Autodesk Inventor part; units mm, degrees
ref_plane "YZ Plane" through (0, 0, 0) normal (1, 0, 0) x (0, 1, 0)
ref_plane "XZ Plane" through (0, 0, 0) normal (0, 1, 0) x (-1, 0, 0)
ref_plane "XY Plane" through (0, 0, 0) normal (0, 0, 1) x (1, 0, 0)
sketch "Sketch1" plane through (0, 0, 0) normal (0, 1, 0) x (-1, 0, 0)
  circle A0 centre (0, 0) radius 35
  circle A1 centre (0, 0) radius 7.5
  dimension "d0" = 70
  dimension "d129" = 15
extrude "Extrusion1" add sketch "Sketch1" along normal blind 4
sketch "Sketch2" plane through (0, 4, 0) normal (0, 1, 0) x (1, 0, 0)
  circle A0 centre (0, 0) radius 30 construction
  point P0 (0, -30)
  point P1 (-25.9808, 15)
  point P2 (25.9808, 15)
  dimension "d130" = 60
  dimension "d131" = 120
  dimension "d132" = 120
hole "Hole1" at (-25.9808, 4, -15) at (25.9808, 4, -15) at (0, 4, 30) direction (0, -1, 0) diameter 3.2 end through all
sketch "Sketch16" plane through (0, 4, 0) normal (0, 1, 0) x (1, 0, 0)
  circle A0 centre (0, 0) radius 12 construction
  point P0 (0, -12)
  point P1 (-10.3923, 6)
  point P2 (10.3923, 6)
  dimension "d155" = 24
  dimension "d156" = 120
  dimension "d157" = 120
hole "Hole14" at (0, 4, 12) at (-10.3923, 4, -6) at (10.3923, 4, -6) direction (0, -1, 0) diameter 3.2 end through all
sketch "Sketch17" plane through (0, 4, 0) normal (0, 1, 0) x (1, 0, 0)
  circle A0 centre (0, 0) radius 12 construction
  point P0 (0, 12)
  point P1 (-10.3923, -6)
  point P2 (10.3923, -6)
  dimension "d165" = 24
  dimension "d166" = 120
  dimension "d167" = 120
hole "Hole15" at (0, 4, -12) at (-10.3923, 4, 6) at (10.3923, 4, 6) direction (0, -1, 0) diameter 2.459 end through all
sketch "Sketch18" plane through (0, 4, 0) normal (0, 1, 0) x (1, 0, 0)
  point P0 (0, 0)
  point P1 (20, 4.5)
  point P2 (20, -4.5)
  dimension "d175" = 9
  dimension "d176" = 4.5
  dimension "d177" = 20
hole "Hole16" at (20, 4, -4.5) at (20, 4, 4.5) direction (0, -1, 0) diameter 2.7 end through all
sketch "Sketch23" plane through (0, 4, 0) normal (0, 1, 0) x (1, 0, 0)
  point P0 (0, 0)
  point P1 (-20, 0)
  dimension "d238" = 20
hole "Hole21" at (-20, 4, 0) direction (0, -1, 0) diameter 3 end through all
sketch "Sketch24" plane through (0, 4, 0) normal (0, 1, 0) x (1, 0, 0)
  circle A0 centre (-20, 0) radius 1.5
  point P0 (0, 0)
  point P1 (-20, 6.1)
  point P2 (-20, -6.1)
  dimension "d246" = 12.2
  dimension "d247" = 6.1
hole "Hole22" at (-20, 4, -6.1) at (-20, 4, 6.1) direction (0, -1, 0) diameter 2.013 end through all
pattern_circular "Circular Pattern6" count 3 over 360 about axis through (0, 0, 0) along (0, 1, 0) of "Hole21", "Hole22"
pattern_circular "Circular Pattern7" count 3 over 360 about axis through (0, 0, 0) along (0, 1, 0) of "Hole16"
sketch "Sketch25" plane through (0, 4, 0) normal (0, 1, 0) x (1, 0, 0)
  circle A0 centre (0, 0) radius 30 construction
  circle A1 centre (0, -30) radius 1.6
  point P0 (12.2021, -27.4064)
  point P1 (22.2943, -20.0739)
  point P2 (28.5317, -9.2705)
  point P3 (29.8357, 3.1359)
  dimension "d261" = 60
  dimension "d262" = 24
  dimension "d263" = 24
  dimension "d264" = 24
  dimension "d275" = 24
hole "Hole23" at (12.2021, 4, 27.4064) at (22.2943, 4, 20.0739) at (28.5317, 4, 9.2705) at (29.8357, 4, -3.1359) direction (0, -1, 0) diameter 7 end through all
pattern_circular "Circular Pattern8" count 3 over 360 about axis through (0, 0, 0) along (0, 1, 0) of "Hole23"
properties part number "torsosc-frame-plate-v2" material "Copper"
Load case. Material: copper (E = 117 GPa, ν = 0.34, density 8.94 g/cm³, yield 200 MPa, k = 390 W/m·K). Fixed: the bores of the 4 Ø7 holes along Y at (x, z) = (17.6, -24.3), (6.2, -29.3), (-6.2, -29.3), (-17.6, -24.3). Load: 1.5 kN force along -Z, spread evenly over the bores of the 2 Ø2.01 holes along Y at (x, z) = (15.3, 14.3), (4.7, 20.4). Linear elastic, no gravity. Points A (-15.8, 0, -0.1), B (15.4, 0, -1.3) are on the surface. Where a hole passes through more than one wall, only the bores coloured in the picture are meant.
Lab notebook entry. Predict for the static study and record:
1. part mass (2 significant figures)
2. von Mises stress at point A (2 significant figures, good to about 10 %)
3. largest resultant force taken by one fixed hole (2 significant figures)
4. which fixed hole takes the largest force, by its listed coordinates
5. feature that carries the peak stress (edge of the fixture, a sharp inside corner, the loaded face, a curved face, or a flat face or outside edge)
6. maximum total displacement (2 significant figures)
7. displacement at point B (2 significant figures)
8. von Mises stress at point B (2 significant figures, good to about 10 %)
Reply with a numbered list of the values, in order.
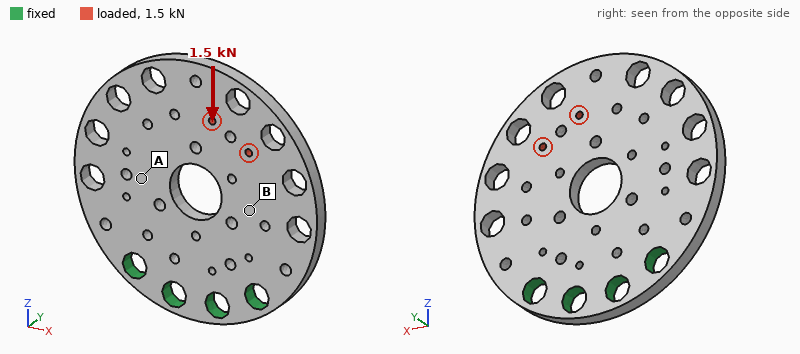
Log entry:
1. 110 g
2. 5.0 MPa
3. 950 N
4. (17.6, -24.3)
5. the loaded face
6. 7.0 µm
7. 3.7 µm
8. 19 MPa
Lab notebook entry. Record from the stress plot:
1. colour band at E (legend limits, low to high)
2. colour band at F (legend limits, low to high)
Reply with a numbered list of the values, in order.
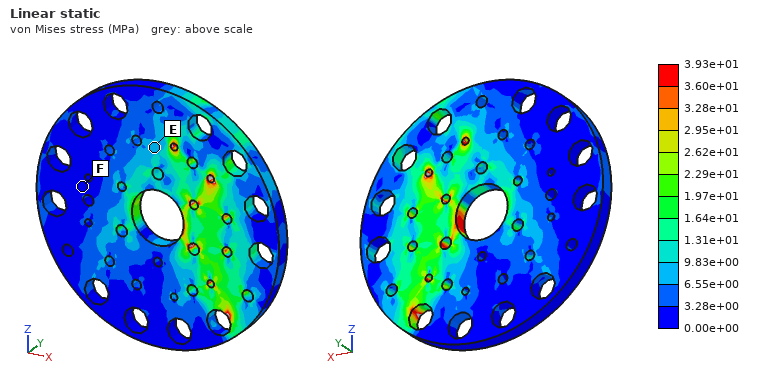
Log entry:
1. 6.55e+00 to 9.83e+00 MPa
2. 0.00e+00 to 3.28e+00 MPa
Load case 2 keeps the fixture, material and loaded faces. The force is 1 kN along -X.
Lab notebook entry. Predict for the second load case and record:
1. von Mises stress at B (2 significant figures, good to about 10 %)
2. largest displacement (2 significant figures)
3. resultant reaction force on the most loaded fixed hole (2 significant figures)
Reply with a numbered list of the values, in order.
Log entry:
1. 16 MPa
2. 16 µm
3. 1.0 kN
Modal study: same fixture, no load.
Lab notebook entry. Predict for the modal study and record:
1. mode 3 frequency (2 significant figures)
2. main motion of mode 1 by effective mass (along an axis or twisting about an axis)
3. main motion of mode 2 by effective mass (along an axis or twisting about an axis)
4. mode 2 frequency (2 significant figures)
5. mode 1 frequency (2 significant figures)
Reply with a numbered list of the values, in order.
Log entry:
1. 3800 Hz
2. along Y
3. twisting about Z
4. 1900 Hz
5. 810 Hz
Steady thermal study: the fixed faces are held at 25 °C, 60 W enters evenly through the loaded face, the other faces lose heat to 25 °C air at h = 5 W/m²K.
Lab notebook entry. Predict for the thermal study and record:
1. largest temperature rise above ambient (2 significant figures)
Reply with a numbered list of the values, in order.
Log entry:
1. 45 K
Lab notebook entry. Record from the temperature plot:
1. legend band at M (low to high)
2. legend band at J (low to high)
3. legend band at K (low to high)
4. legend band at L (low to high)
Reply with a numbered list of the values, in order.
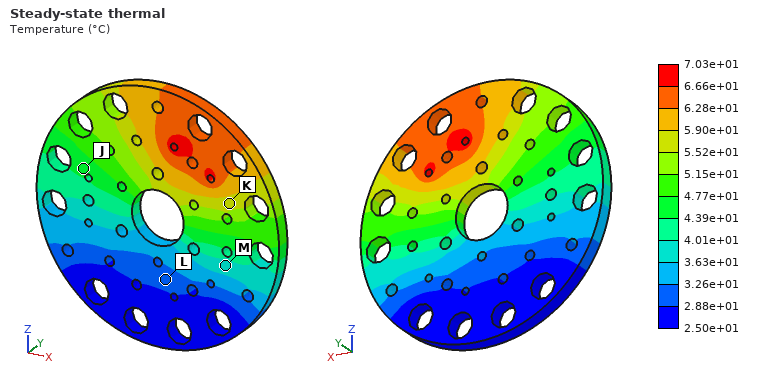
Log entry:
1. 3.63e+01 to 4.01e+01 °C
2. 4.39e+01 to 4.77e+01 °C
3. 5.52e+01 to 5.90e+01 °C
4. 2.88e+01 to 3.26e+01 °C
